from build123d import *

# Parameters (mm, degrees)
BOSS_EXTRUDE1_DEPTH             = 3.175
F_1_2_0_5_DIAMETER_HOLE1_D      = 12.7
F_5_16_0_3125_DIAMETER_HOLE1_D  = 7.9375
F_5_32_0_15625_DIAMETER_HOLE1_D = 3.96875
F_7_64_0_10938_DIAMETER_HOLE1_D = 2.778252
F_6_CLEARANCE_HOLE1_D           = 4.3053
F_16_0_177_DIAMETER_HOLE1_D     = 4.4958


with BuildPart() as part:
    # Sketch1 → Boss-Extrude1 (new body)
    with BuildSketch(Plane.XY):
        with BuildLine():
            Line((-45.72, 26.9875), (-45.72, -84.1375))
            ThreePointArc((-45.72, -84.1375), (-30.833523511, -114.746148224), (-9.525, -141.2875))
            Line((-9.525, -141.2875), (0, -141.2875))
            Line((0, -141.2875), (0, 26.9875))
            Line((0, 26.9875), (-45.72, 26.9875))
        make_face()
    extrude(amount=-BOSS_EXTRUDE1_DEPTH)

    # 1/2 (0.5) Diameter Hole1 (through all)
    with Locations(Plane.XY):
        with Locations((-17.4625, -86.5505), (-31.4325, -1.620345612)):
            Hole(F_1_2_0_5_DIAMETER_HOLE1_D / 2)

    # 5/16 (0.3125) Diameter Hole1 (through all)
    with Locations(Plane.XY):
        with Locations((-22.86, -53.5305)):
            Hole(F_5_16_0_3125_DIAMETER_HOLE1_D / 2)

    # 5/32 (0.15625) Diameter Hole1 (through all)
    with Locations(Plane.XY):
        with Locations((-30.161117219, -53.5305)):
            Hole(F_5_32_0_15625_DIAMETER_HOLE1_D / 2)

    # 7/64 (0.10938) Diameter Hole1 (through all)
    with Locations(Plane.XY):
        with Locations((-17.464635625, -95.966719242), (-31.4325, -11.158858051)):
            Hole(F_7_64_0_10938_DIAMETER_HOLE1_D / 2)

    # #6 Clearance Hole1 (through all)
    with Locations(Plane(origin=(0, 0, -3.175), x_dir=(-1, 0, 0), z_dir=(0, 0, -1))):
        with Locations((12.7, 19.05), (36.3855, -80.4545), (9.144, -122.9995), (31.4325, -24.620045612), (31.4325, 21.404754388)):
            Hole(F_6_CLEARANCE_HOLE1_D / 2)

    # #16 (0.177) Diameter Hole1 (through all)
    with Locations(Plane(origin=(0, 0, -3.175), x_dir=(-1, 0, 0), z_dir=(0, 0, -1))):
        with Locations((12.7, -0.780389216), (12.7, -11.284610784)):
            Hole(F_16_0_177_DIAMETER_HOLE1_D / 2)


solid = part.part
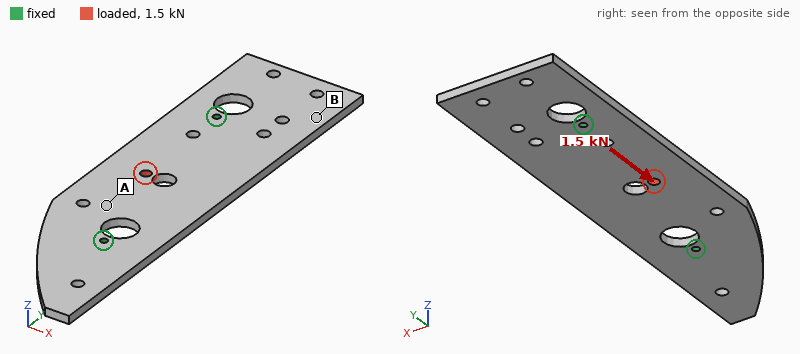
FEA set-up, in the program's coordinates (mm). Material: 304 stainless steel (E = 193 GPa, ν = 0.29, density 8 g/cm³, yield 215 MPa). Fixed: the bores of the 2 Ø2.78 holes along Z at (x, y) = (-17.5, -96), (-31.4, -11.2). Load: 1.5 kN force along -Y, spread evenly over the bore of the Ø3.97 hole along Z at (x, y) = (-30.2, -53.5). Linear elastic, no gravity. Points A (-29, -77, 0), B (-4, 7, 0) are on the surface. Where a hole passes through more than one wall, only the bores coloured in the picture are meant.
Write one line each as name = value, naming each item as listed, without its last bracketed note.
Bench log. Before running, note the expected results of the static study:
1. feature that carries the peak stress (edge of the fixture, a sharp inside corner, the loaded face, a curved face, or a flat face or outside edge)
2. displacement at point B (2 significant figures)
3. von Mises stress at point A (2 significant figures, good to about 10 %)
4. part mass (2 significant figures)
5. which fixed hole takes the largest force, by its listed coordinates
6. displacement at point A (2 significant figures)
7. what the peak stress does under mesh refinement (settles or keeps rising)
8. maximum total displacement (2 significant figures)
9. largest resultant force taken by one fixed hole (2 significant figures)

feature that carries the peak stress = edge of the fixture
displacement at point B = 2.2 µm
von Mises stress at point A = 9.8 MPa
part mass = 160 g
which fixed hole takes the largest force, by its listed coordinates = (-31.4, -11.2)
displacement at point A = 2.5 µm
what the peak stress does under mesh refinement = keeps rising
maximum total displacement = 4.3 µm
largest resultant force taken by one fixed hole = 860 N
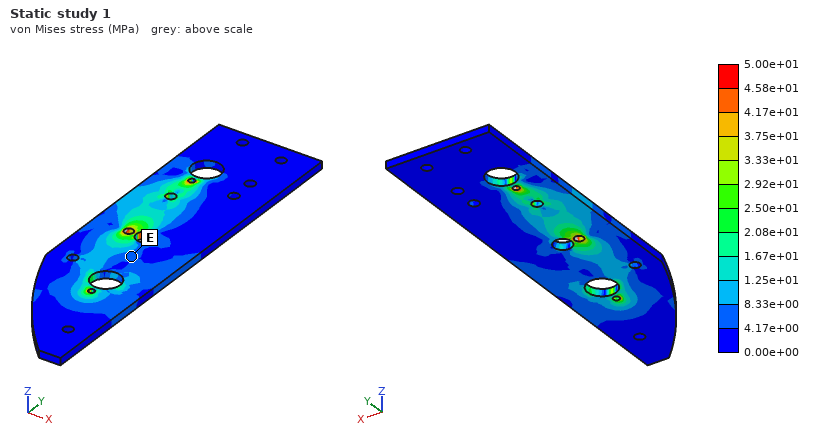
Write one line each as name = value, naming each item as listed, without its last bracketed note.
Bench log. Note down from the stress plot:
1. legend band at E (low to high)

legend band at E = 4.17e+00 to 8.33e+00 MPa
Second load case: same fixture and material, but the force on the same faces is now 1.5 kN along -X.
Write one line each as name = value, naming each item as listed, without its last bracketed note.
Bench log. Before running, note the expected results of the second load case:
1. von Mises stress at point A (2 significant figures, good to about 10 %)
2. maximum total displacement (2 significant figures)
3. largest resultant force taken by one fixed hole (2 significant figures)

von Mises stress at point A = 8.4 MPa
maximum total displacement = 11 µm
largest resultant force taken by one fixed hole = 760 N
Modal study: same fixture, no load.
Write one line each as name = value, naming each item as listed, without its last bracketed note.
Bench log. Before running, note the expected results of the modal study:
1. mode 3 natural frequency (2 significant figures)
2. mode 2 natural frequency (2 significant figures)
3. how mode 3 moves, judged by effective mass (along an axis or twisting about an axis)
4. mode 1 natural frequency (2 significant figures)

mode 3 natural frequency = 1600 Hz
mode 2 natural frequency = 1400 Hz
how mode 3 moves, judged by effective mass = along Z
mode 1 natural frequency = 1000 Hz
